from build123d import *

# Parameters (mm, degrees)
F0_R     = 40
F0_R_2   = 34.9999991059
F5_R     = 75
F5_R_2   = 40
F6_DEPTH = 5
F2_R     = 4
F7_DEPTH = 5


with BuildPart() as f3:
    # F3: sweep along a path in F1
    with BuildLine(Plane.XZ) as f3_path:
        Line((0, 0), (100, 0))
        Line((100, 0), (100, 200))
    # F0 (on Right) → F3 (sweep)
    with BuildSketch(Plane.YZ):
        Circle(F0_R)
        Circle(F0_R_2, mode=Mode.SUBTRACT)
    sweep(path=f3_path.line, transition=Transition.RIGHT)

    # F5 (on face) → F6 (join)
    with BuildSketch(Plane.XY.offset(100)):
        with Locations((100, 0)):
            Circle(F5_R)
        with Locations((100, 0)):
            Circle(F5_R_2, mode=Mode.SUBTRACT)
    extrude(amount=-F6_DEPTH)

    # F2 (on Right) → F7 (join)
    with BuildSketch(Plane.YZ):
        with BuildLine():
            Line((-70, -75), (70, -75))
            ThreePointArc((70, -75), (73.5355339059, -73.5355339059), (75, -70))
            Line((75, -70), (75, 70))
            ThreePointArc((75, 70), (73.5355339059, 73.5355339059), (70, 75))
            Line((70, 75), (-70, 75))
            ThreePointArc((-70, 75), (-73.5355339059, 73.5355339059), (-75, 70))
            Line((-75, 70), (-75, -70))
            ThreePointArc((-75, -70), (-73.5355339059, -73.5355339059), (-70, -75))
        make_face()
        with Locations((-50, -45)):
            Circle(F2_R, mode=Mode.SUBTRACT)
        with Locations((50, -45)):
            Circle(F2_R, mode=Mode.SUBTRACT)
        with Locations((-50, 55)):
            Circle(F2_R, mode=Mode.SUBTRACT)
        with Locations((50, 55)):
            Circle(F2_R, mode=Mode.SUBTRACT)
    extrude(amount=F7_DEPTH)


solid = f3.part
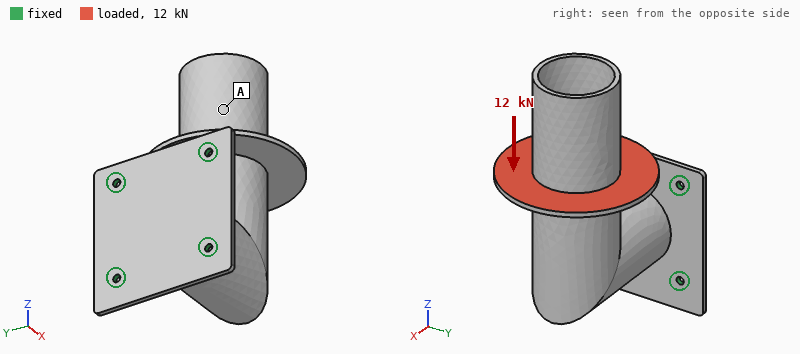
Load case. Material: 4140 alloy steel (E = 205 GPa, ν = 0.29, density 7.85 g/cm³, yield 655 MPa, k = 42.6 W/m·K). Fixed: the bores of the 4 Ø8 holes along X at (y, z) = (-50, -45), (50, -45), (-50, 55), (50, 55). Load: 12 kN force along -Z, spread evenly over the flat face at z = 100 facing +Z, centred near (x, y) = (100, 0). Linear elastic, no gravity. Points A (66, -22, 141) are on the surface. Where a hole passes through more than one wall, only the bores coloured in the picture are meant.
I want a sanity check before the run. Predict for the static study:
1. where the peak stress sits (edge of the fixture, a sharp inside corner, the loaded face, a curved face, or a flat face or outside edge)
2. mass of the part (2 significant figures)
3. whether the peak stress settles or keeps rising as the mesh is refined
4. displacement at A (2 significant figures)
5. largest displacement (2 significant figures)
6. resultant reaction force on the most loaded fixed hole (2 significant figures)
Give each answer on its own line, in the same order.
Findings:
edge of the fixture
4.1 kg
keeps rising
1.1 mm
1.7 mm
7.6 kN
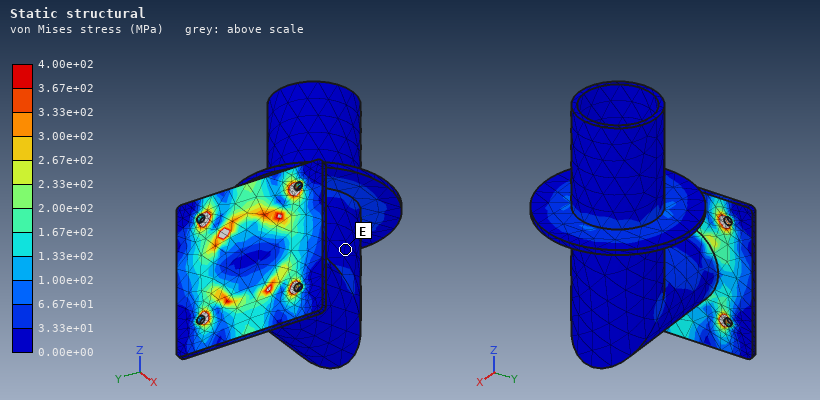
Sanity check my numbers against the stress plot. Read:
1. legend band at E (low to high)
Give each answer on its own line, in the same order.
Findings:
0.00e+00 to 3.33e+01 MPa
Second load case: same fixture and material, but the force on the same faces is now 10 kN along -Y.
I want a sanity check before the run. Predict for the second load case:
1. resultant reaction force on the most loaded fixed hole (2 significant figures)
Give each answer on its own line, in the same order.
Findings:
8.7 kN
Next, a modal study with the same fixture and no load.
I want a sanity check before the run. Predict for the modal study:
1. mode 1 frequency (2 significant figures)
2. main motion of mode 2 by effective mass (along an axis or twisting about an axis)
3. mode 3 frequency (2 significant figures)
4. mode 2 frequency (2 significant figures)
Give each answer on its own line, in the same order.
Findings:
250 Hz
along Y
910 Hz
330 Hz
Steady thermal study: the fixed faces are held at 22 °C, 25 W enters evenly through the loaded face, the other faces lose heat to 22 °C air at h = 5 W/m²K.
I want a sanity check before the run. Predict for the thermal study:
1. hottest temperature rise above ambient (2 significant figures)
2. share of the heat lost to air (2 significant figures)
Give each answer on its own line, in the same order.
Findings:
42 K
76 %
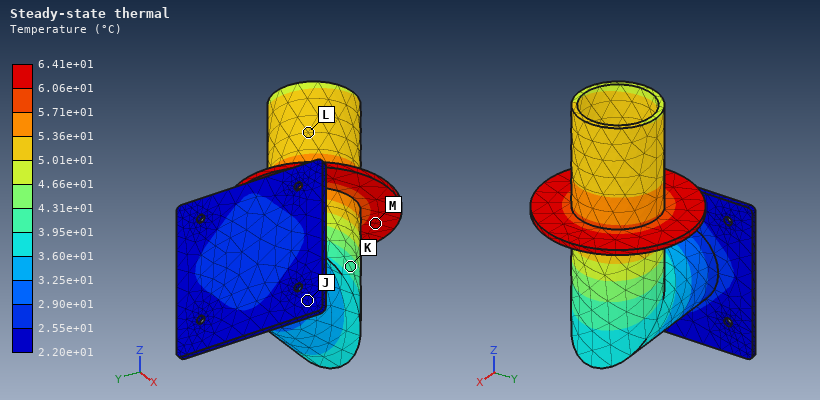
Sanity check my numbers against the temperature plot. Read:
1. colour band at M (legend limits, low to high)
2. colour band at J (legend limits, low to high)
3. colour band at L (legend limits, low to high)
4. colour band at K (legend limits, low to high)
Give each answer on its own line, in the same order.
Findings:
6.06e+01 to 6.41e+01 °C
2.20e+01 to 2.55e+01 °C
5.01e+01 to 5.36e+01 °C
3.95e+01 to 4.31e+01 °C
